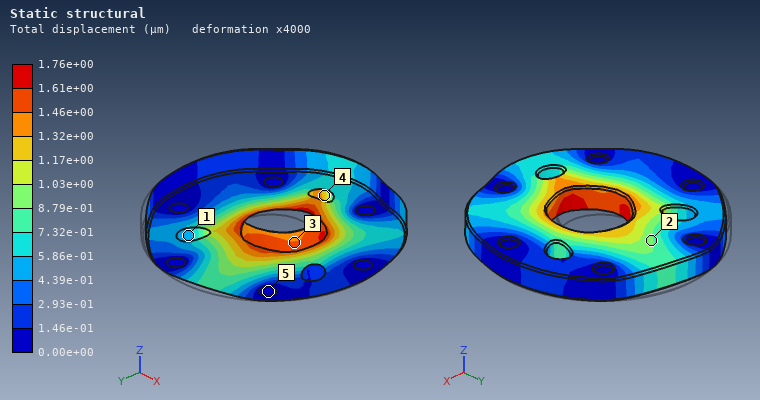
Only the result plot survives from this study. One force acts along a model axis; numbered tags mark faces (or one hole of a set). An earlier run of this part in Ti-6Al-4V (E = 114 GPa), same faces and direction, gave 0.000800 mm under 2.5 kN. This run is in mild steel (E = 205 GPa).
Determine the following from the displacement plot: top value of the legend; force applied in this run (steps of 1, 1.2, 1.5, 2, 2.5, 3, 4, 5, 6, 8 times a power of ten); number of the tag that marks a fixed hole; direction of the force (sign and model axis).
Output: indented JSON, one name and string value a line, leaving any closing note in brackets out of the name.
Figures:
{
  "top value of the legend": "1.76e+00 µm",
  "force applied in this run": "10 kN",
  "number of the tag that marks a fixed hole": "5",
  "direction of the force": "-Y"
}
